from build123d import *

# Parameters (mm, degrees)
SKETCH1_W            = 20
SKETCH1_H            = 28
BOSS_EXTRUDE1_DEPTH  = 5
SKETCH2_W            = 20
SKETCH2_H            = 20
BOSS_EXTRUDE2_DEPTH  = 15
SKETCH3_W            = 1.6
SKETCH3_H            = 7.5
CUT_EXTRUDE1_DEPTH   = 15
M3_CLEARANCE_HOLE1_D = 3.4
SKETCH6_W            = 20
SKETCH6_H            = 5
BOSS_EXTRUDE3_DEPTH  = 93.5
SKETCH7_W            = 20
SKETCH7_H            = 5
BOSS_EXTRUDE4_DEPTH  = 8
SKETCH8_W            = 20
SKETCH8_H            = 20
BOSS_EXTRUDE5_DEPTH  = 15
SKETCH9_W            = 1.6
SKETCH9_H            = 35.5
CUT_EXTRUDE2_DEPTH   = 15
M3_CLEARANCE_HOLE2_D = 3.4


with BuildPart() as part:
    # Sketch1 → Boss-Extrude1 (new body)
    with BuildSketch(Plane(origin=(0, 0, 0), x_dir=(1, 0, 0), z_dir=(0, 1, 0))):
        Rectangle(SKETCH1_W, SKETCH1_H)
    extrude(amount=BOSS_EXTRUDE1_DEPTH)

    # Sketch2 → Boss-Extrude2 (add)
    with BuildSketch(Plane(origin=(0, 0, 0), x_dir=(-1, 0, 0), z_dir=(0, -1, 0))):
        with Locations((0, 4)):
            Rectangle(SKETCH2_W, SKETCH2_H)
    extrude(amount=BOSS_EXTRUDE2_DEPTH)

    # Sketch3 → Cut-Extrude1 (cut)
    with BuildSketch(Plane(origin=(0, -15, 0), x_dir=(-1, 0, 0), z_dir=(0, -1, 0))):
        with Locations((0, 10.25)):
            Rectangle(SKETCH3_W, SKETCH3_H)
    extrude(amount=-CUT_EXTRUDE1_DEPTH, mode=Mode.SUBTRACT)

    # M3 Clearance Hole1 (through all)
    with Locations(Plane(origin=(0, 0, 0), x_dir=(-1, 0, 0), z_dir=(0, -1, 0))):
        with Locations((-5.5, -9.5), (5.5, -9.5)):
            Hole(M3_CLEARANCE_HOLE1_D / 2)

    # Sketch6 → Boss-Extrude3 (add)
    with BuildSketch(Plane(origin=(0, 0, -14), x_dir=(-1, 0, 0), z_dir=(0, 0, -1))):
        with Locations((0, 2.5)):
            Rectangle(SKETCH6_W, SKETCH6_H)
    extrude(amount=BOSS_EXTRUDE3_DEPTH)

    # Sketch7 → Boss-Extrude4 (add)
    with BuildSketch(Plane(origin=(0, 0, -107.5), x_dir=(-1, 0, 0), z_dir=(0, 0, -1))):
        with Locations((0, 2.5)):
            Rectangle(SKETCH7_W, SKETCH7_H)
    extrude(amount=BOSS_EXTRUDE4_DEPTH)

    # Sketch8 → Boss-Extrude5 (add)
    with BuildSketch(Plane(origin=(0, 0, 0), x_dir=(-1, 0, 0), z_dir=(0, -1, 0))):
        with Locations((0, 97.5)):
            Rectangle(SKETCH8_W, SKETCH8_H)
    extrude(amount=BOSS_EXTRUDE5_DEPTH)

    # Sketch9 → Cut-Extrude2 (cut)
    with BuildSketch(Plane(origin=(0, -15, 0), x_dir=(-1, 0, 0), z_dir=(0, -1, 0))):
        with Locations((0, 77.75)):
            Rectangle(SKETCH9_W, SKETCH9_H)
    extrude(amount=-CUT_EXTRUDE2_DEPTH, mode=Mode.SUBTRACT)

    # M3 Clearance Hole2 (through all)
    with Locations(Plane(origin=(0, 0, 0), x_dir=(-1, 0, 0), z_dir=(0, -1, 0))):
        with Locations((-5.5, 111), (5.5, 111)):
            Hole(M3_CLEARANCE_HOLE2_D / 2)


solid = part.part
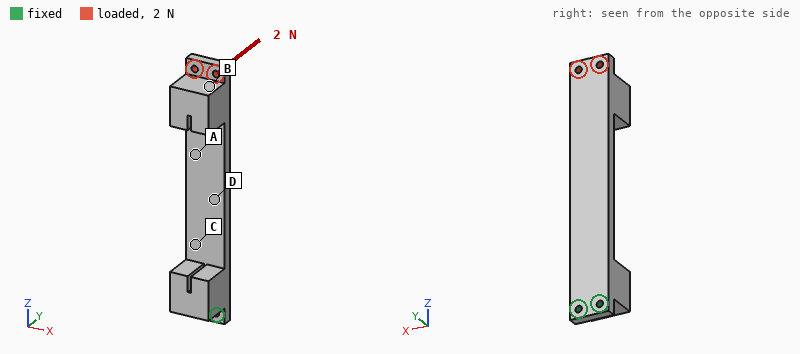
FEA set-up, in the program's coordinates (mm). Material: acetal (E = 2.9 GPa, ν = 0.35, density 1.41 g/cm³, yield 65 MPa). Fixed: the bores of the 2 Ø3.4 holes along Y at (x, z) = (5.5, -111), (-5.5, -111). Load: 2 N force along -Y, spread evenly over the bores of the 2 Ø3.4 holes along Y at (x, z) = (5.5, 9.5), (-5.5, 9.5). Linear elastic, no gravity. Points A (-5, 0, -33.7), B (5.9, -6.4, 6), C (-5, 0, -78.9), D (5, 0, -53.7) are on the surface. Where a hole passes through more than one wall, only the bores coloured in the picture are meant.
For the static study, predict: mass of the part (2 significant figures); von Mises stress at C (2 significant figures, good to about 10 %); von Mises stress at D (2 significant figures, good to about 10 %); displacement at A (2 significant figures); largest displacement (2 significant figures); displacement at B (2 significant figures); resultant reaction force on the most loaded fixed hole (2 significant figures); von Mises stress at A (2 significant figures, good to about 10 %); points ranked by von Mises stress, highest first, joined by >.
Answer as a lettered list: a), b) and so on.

a) 34 g
b) 2.0 MPa
c) 1.5 MPa
d) 0.59 mm
e) 1.4 mm
f) 1.3 mm
g) 1.0 N
h) 1.0 MPa
i) C > D > A > B
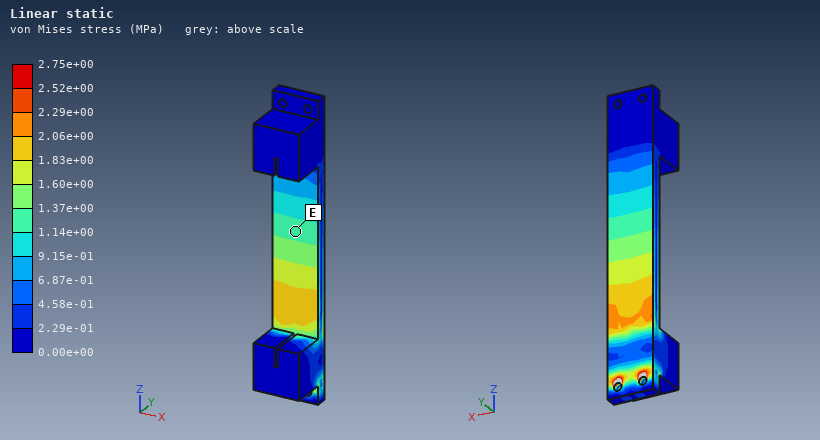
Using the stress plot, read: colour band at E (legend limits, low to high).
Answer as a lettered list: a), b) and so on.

a) 1.14e+00 to 1.37e+00 MPa
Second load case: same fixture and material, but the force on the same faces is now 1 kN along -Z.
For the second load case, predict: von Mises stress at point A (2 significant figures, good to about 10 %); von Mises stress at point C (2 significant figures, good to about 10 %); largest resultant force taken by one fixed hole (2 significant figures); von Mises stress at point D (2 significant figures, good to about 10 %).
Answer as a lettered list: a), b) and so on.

a) 10.0 MPa
b) 9.9 MPa
c) 500 N
d) 10.0 MPa
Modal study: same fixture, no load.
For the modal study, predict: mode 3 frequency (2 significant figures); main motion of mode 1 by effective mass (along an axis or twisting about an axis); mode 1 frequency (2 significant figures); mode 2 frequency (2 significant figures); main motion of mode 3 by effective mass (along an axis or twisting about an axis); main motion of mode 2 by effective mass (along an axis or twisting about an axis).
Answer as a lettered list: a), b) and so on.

a) 430 Hz
b) along Y
c) 61 Hz
d) 200 Hz
e) along Y
f) along X
